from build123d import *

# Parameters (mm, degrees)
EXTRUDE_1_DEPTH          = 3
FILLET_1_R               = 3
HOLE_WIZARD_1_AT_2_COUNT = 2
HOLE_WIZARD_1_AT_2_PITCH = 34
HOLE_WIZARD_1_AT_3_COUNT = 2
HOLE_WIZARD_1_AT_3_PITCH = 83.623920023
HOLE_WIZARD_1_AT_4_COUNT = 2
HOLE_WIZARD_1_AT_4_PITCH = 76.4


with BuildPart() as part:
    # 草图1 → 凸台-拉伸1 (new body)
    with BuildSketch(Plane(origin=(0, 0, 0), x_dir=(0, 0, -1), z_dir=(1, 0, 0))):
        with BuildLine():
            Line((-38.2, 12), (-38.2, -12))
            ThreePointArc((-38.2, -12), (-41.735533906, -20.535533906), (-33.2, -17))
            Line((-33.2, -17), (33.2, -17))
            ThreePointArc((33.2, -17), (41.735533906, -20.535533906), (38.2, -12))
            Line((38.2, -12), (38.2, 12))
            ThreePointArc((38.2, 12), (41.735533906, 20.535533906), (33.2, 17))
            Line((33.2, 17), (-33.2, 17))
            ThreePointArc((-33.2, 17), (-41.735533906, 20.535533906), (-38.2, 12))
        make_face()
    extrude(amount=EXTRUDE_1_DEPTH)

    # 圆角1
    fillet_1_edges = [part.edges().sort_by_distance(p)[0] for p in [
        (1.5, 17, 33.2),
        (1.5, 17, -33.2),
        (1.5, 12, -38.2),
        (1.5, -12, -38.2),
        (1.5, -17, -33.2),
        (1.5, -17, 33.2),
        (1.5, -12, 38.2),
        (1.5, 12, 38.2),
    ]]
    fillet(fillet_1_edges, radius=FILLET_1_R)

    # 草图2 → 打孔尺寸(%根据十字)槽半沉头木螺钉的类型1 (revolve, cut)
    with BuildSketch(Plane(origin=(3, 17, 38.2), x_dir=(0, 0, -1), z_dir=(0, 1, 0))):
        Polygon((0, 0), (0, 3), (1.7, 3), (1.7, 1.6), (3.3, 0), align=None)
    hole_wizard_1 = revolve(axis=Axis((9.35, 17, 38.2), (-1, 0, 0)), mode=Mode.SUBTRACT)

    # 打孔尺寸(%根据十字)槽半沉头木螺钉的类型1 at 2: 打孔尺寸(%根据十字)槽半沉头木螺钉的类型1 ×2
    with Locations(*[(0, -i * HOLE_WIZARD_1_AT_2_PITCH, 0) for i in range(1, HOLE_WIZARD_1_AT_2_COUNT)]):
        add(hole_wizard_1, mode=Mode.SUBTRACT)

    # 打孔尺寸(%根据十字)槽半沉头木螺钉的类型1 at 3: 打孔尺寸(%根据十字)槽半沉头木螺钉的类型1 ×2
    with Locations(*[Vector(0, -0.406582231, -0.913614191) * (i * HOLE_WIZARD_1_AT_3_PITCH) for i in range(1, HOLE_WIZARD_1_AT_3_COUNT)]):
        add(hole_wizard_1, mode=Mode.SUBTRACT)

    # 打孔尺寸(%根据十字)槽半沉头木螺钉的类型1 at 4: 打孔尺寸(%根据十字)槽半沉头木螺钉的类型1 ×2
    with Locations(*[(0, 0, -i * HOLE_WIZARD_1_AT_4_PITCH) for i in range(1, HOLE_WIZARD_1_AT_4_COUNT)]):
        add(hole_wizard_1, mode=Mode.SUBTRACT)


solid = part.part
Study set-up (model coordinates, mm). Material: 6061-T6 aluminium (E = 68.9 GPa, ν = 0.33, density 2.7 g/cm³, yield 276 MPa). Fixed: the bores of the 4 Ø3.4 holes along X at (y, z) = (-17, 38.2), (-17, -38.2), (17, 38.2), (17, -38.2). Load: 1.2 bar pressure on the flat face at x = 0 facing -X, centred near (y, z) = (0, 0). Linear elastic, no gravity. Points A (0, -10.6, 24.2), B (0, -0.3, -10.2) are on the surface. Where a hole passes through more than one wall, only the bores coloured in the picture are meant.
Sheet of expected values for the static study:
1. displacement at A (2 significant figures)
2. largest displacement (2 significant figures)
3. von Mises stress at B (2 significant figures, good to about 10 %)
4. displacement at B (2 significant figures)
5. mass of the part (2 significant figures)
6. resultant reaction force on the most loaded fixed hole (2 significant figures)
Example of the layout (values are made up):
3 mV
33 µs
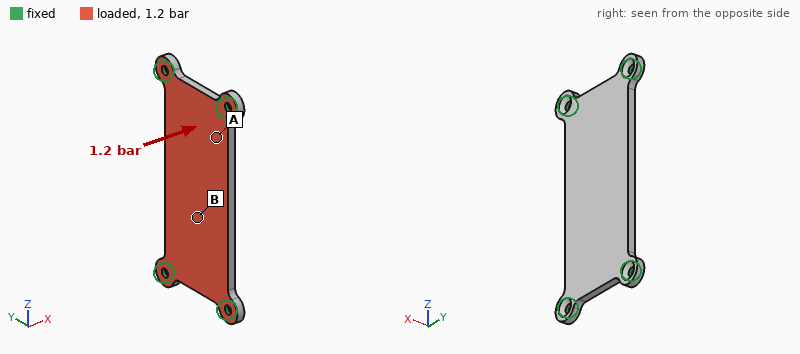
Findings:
0.053 mm
0.12 mm
18 MPa
0.10 mm
23 g
140 N
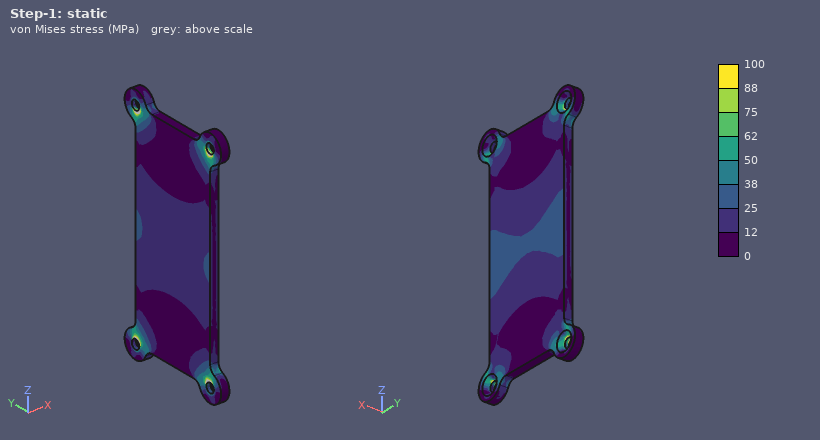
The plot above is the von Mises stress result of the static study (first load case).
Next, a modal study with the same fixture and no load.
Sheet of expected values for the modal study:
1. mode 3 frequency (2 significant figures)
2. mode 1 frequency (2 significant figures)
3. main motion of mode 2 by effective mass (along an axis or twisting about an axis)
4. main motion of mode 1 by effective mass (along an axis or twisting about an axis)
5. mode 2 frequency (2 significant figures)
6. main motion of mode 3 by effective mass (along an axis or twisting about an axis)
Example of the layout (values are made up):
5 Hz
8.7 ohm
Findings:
5800 Hz
2100 Hz
twisting about Z
along X
4500 Hz
twisting about Y
